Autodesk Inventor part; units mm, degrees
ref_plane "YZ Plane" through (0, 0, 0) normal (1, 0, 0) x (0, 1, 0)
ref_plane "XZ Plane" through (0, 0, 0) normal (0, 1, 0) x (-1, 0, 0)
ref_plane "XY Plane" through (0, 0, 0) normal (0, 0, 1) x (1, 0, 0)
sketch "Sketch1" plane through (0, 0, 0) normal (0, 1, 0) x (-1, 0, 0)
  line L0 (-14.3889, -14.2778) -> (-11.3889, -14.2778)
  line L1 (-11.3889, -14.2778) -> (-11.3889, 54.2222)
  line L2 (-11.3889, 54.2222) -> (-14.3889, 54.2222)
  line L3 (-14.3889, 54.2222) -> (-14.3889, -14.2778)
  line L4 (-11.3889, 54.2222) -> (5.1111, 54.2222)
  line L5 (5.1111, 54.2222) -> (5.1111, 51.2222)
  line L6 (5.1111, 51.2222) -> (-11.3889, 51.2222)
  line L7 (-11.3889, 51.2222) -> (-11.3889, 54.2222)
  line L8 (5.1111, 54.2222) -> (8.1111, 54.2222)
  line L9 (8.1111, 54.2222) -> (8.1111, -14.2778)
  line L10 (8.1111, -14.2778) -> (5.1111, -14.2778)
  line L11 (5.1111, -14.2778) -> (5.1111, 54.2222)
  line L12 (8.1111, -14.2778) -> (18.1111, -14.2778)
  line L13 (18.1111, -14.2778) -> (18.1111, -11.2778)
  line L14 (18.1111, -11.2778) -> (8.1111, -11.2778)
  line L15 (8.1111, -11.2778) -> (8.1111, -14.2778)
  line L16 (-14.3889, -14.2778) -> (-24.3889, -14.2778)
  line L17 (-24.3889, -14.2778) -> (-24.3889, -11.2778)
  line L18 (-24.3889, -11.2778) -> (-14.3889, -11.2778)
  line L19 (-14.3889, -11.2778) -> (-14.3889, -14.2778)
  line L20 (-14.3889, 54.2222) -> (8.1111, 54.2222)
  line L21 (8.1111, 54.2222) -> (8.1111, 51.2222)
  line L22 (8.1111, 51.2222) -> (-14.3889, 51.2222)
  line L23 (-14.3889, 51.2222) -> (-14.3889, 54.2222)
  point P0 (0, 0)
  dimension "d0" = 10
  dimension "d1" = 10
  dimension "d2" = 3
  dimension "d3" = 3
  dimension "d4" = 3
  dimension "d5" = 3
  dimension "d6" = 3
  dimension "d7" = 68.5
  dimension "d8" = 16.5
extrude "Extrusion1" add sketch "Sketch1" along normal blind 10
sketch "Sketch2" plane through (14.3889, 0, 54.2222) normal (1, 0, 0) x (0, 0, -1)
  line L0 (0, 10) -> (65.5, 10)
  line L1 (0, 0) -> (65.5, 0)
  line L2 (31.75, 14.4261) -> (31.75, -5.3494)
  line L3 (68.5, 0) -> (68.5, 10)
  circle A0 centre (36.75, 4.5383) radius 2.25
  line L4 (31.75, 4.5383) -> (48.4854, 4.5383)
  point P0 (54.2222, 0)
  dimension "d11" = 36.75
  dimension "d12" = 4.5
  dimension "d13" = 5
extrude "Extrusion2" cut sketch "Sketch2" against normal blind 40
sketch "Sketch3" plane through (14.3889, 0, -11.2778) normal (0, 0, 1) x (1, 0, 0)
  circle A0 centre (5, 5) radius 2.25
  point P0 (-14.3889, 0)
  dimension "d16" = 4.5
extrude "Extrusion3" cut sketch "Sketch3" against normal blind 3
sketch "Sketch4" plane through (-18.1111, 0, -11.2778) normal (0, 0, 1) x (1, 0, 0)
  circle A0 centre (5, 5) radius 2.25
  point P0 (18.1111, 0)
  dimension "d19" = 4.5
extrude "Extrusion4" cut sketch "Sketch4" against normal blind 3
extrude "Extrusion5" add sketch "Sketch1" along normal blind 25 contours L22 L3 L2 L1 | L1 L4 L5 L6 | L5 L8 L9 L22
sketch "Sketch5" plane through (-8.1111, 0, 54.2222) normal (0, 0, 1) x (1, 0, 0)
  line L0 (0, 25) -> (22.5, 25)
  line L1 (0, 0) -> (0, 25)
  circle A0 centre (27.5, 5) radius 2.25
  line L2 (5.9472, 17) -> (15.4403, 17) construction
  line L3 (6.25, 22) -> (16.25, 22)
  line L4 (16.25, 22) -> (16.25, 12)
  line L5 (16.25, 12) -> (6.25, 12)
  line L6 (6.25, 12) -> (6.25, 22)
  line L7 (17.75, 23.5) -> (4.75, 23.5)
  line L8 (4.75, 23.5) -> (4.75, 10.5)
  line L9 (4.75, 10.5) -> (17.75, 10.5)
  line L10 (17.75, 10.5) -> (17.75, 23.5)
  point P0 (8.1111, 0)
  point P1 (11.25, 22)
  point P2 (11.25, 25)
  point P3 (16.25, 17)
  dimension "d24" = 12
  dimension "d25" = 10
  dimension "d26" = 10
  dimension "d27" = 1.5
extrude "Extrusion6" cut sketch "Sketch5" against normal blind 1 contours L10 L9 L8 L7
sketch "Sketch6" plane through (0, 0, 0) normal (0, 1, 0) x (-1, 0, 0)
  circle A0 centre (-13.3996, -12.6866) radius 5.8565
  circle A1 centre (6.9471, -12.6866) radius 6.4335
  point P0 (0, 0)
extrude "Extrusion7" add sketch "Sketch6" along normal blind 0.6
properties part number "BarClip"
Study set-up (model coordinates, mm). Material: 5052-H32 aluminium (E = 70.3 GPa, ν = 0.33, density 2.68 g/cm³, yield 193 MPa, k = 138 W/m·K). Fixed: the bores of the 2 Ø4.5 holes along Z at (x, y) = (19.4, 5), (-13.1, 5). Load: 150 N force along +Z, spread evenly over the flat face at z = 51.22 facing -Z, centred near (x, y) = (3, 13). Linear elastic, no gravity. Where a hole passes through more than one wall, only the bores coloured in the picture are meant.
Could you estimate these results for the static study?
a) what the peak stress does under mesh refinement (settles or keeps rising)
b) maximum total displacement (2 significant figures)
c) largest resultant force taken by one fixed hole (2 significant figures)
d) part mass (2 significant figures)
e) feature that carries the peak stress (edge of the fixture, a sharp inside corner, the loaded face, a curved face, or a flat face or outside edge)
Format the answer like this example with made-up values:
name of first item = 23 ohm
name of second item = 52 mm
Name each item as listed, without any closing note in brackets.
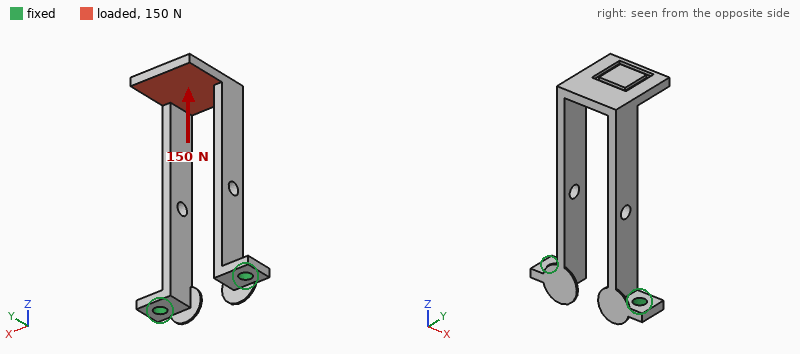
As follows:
what the peak stress does under mesh refinement = keeps rising
maximum total displacement = 0.18 mm
largest resultant force taken by one fixed hole = 75 N
part mass = 16 g
feature that carries the peak stress = edge of the fixture
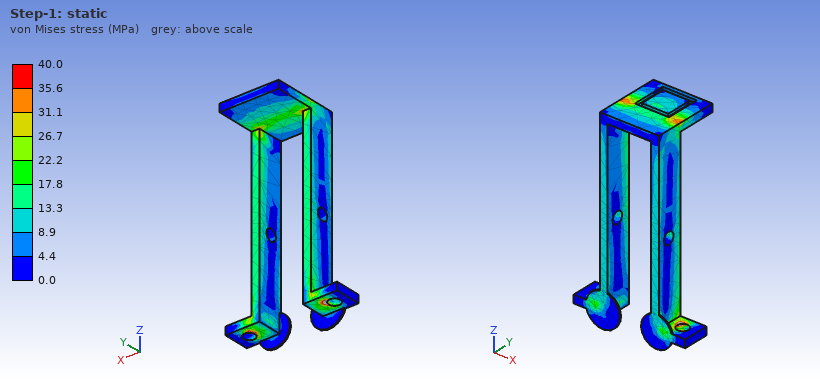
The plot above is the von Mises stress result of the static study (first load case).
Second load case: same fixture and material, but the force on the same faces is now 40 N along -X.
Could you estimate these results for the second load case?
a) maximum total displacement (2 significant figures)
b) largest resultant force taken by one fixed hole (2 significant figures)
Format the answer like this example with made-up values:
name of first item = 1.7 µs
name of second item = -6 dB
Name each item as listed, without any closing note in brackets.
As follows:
maximum total displacement = 0.39 mm
largest resultant force taken by one fixed hole = 67 N
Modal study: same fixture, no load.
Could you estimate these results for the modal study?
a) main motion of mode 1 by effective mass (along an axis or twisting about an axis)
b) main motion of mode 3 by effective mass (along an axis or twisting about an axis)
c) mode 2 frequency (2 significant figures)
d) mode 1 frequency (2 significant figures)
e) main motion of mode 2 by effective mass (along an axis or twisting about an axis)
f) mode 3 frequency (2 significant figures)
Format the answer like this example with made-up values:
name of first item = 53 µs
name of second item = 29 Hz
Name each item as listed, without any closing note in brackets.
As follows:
main motion of mode 1 by effective mass = along X
main motion of mode 3 by effective mass = twisting about Z
mode 2 frequency = 790 Hz
mode 1 frequency = 630 Hz
main motion of mode 2 by effective mass = along Y
mode 3 frequency = 1600 Hz
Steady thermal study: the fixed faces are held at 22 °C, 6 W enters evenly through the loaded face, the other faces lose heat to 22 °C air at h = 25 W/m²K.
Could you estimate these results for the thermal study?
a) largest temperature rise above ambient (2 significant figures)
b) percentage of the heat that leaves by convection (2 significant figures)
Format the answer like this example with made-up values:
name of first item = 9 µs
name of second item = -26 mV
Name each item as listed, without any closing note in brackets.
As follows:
largest temperature rise above ambient = 41 K
percentage of the heat that leaves by convection = 40 %
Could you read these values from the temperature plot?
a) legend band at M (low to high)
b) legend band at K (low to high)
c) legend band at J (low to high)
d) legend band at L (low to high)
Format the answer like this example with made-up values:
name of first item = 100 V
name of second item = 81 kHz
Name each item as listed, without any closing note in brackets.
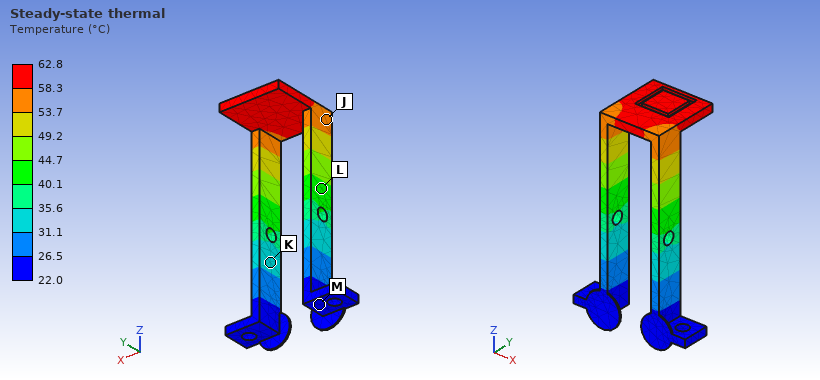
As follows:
legend band at M = 22.0 to 26.5 °C
legend band at K = 31.1 to 35.6 °C
legend band at J = 53.7 to 58.3 °C
legend band at L = 40.1 to 44.7 °C
